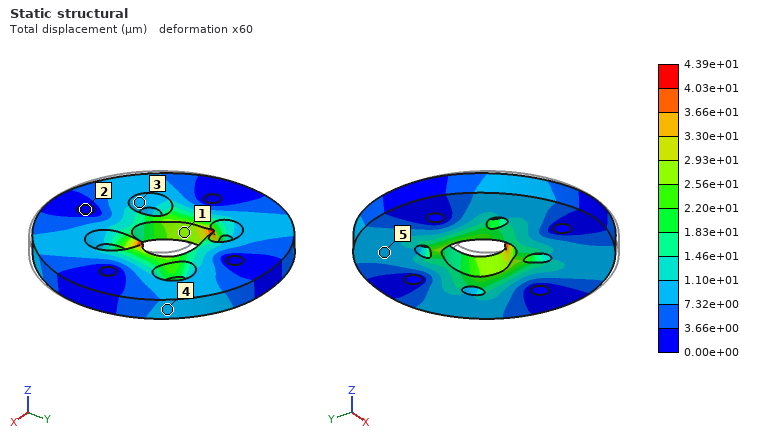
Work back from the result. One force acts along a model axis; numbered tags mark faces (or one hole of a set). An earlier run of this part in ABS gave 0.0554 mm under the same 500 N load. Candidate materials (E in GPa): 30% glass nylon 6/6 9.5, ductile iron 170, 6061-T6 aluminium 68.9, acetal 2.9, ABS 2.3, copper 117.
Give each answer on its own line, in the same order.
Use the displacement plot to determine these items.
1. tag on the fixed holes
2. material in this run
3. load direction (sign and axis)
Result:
2
acetal
+Y
